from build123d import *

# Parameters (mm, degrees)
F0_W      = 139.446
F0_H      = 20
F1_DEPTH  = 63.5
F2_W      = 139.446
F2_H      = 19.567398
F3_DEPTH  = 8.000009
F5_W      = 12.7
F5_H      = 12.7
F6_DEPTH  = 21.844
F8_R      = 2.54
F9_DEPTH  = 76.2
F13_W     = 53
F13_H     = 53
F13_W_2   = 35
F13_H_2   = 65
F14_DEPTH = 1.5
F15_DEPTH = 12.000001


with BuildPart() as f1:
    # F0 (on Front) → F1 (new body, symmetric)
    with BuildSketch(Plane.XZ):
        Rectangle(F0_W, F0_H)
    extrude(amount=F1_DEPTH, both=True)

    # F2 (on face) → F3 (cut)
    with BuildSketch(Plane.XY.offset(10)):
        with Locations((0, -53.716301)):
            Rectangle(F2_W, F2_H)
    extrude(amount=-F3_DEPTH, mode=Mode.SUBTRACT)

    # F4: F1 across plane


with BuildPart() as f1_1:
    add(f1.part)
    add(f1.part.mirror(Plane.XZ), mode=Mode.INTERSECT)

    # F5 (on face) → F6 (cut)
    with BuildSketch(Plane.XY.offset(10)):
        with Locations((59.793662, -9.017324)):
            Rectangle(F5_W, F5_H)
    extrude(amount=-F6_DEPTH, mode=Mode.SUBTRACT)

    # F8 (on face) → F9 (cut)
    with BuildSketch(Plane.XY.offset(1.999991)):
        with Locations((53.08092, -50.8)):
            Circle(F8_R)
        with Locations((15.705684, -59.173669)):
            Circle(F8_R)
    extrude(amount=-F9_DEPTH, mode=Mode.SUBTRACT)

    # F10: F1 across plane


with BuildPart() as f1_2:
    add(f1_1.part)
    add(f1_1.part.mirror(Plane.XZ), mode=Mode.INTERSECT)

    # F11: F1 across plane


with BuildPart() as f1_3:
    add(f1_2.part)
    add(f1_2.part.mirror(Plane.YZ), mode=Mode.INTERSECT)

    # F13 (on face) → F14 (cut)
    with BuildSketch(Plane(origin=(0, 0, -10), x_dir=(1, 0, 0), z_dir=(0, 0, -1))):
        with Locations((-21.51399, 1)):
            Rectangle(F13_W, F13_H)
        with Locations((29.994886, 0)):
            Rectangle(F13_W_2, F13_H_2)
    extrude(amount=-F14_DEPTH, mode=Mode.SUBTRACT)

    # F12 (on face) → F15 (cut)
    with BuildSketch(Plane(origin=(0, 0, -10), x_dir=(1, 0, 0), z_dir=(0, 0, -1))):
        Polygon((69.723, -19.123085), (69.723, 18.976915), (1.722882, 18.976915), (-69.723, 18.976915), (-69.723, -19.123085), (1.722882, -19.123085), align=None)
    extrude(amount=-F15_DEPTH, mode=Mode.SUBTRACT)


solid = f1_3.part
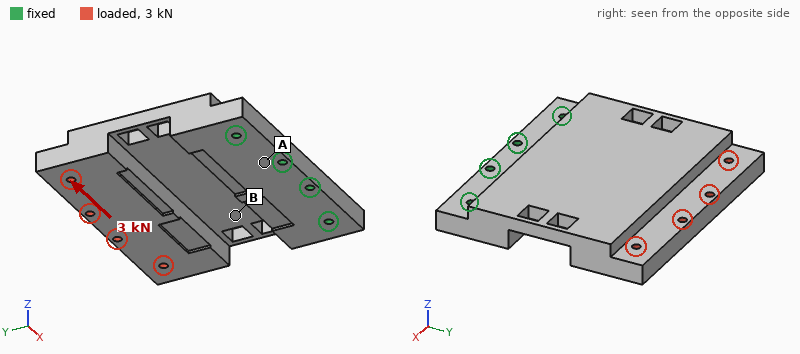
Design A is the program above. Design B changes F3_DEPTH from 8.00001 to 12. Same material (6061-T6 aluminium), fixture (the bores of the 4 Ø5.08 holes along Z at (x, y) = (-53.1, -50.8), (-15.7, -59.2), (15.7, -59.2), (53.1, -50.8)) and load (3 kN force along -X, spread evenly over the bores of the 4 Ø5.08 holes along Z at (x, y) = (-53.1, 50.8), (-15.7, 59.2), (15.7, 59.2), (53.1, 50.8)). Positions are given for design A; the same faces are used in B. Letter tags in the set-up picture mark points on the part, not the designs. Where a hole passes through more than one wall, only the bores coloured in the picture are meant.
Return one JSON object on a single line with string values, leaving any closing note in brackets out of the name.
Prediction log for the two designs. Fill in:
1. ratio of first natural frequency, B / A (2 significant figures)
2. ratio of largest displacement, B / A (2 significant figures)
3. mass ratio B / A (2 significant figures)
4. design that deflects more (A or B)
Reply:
{"ratio of first natural frequency, B / A": "0.85", "ratio of largest displacement, B / A": "1.6", "mass ratio B / A": "0.91", "design that deflects more": "B"}
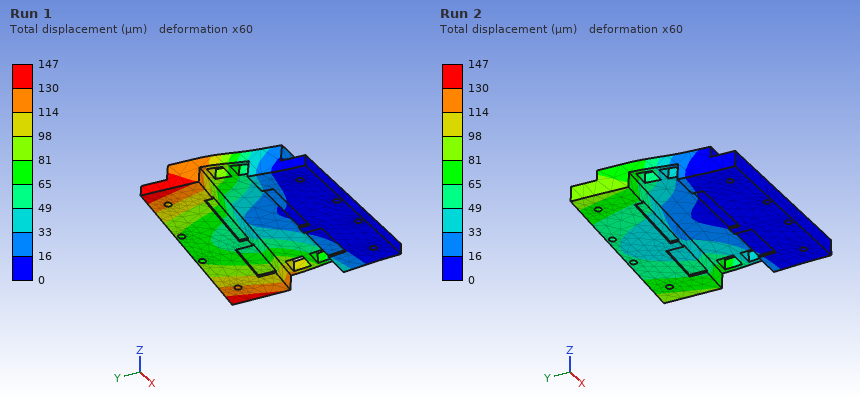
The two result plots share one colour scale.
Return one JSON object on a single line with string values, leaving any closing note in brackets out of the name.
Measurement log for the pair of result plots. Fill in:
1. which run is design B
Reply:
{"which run is design B": "Run 1"}
